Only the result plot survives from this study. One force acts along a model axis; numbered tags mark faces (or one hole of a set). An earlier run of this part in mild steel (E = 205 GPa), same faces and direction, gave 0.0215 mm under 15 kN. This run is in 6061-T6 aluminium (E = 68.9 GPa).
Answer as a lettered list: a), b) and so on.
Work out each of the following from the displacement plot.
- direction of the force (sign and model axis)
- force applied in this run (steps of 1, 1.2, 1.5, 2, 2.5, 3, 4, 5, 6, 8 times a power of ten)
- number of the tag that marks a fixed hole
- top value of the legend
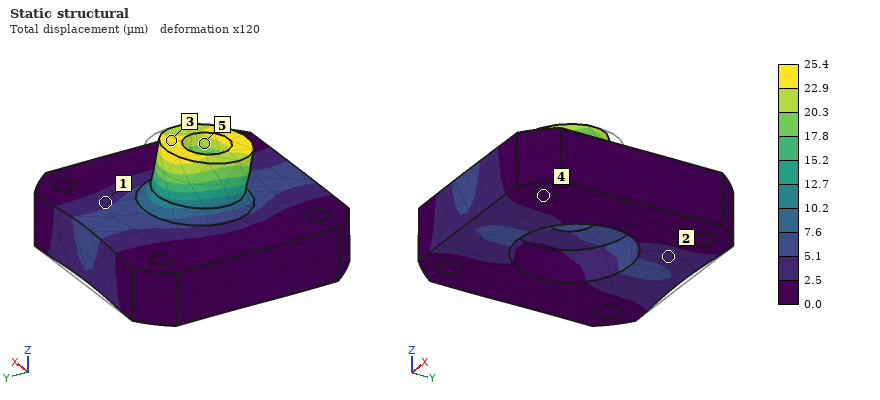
a) -Y
b) 6 kN
c) 4
d) 25.4 µm
